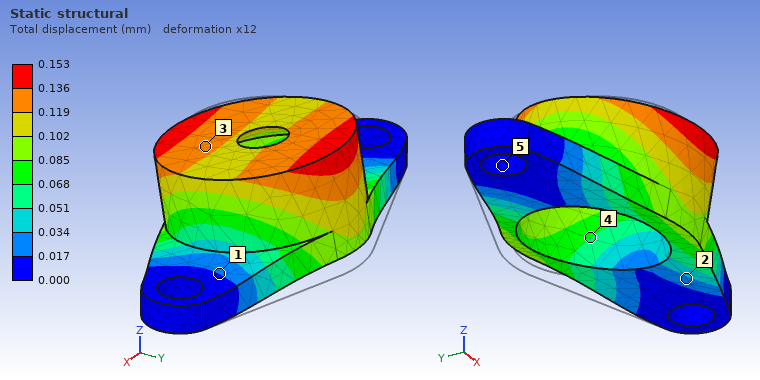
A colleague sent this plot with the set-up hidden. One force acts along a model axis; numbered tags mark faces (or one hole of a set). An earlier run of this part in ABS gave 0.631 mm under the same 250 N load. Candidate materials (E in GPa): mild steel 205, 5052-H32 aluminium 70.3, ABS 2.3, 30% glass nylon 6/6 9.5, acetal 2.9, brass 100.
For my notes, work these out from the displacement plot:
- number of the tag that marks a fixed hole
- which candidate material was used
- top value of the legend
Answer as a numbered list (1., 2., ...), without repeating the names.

1. 5
2. 30% glass nylon 6/6
3. 0.153 mm
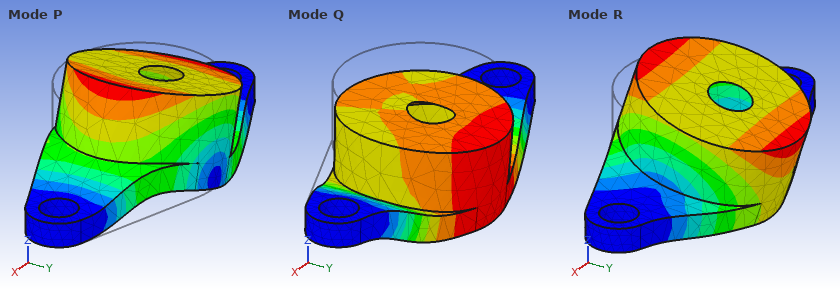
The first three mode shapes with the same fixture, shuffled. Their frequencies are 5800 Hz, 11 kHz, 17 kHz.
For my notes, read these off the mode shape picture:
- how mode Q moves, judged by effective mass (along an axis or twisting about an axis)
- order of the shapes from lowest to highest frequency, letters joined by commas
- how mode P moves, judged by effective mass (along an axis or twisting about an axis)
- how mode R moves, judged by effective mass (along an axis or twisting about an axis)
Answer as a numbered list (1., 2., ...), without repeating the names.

1. along Z
2. R, Q, P
3. along X
4. along Y
